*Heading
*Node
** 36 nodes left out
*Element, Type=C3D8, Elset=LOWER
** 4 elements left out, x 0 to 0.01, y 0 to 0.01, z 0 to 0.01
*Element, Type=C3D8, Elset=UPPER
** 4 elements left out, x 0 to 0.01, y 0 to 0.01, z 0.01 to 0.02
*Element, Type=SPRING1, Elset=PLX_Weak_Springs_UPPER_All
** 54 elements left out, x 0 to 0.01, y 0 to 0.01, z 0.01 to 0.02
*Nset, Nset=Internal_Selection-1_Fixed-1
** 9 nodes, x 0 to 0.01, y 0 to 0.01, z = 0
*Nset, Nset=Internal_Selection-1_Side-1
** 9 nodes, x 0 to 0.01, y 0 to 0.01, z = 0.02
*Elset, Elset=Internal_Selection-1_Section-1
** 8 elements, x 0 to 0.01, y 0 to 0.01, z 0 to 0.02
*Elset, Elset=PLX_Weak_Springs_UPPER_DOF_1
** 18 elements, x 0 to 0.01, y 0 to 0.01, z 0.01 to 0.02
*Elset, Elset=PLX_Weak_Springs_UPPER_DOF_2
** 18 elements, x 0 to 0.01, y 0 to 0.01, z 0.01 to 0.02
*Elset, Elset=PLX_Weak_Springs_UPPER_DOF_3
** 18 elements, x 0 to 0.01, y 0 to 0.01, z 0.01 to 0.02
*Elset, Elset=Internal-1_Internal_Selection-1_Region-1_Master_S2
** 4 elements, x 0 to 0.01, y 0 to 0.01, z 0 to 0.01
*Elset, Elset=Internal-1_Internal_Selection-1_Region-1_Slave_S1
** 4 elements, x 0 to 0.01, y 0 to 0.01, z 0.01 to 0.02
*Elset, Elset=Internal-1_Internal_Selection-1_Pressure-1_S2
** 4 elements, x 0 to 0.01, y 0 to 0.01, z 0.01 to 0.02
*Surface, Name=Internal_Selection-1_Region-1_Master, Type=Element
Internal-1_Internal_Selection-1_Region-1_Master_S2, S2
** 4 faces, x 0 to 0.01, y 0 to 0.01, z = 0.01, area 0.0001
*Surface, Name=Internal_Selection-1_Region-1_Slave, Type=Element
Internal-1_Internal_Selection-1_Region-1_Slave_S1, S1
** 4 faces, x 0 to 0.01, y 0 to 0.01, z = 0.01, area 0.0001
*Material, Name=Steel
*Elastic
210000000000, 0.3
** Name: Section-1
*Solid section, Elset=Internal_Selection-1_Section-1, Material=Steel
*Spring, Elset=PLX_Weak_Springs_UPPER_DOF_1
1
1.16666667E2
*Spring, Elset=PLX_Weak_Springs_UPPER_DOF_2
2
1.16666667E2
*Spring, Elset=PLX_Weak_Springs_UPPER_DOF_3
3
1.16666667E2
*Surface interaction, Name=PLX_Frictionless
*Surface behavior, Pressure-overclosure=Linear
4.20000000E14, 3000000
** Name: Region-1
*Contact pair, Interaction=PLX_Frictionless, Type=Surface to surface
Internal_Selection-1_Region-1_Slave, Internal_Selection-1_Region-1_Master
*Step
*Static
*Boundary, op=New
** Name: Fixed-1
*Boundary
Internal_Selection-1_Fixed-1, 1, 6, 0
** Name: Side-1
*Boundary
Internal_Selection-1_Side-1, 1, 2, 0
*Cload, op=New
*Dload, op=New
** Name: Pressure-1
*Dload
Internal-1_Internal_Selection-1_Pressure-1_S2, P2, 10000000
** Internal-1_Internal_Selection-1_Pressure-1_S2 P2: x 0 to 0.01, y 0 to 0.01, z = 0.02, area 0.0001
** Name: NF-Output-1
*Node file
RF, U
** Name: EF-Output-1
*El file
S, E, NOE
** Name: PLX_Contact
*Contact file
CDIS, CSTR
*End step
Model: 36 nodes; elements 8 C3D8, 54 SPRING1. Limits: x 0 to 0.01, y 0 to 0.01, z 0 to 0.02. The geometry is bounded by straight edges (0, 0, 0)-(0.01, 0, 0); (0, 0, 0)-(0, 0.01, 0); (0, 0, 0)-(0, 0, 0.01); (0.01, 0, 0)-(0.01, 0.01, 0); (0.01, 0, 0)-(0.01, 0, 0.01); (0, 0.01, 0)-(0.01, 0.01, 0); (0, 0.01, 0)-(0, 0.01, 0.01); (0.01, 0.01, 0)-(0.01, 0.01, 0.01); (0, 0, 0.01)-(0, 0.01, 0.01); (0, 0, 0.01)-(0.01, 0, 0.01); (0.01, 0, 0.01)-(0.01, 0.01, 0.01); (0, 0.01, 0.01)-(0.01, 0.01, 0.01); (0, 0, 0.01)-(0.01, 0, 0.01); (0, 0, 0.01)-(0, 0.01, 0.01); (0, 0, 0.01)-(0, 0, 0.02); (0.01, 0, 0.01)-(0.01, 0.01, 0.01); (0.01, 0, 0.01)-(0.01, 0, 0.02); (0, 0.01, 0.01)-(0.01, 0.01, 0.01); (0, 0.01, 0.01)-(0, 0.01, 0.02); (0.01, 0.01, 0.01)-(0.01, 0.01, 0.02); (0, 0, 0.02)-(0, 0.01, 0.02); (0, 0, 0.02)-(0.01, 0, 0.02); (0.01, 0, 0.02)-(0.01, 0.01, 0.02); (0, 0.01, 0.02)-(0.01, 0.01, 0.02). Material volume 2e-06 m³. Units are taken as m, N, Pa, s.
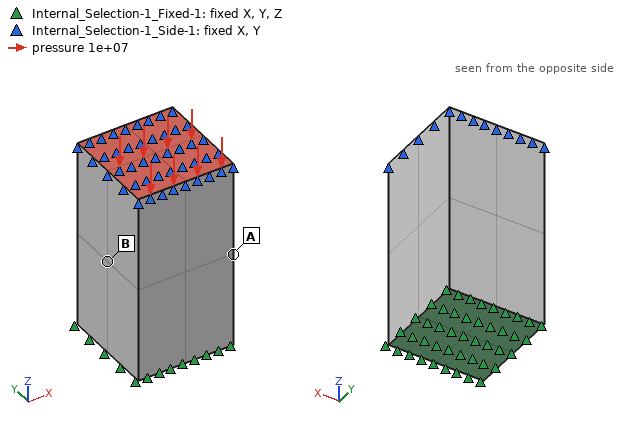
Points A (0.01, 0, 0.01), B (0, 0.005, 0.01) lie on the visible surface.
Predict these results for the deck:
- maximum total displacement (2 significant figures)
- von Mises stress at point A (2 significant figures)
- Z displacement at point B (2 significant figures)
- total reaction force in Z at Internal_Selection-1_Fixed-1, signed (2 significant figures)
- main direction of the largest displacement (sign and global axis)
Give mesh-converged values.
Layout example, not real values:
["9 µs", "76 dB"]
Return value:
["9.7e-07 m", "9.6e+06 Pa", "-4.6e-07 m", "1000 N", "-Z"]
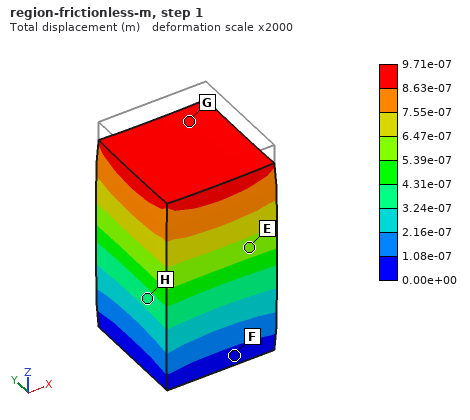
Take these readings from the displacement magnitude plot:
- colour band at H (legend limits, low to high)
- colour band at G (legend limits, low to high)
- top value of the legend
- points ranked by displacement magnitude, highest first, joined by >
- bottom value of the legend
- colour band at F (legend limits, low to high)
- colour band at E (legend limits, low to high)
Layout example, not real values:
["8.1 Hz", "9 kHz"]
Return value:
["3.24e-07 to 4.31e-07 m", "8.63e-07 to 9.71e-07 m", "9.71e-07 m", "G > E > H > F", "0.00e+00 m", "0.00e+00 to 1.08e-07 m", "5.39e-07 to 6.47e-07 m"]
